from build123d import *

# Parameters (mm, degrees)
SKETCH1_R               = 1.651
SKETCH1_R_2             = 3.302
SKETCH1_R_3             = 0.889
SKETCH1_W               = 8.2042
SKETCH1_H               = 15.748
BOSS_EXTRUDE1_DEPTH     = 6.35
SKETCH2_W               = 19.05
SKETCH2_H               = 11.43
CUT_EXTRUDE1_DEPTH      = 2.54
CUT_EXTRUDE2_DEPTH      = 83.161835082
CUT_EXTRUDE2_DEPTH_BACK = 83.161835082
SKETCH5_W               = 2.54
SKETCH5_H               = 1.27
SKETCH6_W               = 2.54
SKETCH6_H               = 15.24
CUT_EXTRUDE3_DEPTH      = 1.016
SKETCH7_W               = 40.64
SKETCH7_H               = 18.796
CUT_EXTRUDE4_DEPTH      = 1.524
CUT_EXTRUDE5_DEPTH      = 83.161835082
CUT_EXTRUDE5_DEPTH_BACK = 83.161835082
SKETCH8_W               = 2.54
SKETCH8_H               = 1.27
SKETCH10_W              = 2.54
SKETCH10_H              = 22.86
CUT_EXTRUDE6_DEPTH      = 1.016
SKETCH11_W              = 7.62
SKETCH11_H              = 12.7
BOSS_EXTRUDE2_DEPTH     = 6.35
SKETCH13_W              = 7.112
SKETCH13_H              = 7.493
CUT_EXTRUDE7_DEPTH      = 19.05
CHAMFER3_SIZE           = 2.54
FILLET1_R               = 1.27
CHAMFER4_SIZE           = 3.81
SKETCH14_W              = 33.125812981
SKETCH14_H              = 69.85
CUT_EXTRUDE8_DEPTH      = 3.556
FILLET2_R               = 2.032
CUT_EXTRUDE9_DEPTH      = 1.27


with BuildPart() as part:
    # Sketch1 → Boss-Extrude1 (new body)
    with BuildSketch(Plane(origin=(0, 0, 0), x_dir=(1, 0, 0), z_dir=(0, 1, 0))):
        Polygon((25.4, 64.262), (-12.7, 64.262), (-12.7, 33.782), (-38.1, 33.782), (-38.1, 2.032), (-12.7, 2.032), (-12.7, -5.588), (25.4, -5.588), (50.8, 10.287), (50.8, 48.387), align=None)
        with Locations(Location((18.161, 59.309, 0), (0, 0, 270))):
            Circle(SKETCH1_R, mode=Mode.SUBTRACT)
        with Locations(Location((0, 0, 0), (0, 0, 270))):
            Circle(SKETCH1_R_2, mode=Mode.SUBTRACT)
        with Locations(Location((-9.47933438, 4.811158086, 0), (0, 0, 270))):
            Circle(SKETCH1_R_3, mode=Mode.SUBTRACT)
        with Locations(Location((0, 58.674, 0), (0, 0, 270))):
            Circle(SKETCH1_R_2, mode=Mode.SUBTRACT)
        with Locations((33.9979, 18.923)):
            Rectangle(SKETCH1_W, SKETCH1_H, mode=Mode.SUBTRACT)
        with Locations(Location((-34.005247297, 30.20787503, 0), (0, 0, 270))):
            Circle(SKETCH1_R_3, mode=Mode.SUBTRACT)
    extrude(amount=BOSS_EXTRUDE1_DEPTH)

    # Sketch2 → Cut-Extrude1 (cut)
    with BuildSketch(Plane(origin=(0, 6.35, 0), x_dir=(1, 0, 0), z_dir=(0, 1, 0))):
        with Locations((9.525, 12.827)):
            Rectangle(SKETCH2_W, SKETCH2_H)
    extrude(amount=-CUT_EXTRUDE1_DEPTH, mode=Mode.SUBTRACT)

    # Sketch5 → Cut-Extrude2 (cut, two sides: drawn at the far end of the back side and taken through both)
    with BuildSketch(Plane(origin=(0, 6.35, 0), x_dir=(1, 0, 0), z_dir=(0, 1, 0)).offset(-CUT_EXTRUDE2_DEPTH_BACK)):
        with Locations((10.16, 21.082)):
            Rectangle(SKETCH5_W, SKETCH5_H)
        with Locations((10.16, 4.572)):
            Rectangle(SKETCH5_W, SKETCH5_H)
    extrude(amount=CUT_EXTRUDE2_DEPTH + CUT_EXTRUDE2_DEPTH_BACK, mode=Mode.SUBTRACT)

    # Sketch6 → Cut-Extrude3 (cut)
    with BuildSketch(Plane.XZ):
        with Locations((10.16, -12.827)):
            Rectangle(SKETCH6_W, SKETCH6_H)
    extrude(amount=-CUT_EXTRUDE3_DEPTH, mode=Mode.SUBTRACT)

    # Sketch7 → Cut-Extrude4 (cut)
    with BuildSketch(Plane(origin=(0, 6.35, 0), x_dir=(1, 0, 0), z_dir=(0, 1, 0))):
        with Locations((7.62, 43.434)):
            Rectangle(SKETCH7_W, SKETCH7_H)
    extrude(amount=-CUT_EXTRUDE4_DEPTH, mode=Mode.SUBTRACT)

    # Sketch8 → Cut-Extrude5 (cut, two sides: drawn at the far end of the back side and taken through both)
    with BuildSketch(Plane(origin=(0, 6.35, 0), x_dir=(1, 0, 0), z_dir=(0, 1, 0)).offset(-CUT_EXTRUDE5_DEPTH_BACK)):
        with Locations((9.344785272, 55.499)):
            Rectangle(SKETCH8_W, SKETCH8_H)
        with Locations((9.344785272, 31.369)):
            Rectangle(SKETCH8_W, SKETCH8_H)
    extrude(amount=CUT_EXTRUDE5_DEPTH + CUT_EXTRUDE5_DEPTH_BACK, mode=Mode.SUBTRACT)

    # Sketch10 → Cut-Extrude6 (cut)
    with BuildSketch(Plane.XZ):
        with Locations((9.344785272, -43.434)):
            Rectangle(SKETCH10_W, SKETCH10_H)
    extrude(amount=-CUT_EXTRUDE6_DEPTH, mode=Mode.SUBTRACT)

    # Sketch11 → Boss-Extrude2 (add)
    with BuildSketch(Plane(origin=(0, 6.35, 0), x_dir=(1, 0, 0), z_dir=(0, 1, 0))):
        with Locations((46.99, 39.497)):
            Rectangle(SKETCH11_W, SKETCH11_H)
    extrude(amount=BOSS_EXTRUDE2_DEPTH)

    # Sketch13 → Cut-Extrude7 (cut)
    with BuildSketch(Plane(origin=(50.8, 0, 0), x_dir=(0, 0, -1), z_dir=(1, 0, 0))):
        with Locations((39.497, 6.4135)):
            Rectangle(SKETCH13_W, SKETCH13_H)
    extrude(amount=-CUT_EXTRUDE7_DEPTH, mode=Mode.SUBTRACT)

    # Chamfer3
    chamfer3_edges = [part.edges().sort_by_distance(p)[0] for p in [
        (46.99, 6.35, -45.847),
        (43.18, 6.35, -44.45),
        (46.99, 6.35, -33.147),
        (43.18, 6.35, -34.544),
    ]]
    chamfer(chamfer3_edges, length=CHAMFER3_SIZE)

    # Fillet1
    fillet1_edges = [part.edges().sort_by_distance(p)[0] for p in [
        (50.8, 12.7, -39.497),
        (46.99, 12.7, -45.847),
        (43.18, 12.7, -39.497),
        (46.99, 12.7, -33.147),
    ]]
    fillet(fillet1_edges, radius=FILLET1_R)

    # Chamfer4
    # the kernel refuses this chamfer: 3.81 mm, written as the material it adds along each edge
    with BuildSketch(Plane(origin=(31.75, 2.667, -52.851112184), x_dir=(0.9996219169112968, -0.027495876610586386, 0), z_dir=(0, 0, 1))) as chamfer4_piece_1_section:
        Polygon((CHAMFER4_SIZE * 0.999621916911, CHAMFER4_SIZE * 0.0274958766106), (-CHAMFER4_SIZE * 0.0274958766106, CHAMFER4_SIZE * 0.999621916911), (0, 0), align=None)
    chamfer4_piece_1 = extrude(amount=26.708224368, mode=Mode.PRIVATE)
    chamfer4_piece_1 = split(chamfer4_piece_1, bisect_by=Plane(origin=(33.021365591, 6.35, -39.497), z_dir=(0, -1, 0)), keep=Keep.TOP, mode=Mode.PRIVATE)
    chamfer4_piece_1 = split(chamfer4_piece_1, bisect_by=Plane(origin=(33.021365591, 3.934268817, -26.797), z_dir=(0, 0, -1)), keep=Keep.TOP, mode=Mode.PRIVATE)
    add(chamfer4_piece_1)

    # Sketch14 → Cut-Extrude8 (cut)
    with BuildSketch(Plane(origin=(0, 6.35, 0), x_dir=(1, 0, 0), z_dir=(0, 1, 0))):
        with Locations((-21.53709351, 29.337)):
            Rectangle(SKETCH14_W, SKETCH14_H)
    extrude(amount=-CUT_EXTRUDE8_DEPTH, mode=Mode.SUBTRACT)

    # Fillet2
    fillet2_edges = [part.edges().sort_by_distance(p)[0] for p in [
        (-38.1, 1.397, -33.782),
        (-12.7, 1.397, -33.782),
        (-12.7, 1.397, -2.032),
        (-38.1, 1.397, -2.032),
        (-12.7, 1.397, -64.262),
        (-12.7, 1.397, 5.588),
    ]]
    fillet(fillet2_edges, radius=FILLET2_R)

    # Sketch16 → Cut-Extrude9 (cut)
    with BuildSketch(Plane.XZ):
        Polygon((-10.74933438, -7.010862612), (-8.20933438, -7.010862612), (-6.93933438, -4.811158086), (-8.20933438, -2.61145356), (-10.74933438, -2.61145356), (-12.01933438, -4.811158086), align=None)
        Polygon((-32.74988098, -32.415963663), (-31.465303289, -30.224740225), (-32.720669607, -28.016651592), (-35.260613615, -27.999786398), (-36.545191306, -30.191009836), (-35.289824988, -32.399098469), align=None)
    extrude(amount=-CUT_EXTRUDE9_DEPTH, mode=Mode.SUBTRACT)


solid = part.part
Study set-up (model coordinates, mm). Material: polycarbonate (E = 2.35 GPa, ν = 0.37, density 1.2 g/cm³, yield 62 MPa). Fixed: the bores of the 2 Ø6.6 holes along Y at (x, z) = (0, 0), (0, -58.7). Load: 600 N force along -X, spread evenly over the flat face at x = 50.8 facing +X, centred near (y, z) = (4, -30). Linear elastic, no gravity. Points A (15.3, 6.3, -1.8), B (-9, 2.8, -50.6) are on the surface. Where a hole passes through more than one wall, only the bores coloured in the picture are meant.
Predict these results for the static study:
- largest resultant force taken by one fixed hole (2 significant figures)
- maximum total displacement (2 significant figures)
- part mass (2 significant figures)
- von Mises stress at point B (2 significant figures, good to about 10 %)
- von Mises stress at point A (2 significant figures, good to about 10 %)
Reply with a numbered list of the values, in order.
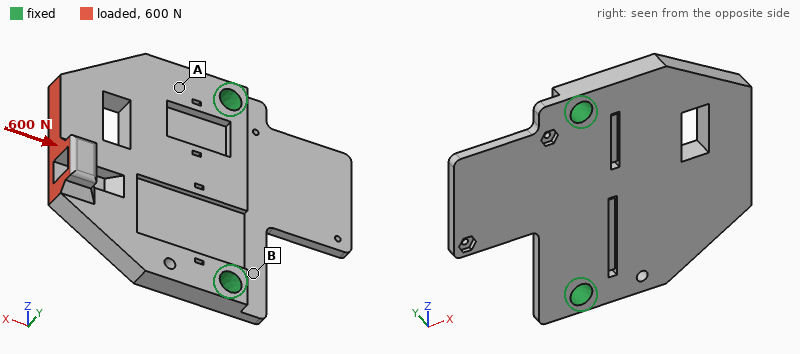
1. 320 N
2. 0.48 mm
3. 28 g
4. 1.6 MPa
5. 4.8 MPa
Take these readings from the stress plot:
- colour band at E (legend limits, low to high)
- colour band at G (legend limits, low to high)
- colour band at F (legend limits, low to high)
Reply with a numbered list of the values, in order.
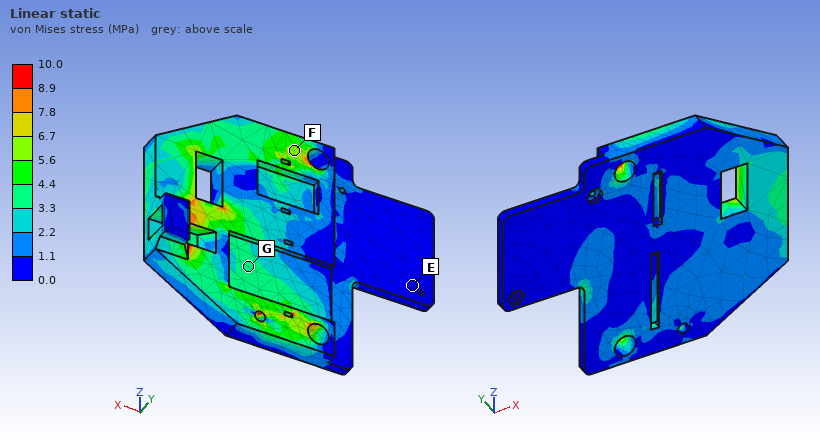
1. 0.0 to 1.1 MPa
2. 3.3 to 4.4 MPa
3. 5.6 to 6.7 MPa
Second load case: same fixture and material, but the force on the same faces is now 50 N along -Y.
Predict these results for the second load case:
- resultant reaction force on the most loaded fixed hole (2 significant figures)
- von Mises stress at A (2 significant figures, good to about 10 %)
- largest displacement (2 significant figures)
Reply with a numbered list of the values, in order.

1. 26 N
2. 6.9 MPa
3. 1.2 mm
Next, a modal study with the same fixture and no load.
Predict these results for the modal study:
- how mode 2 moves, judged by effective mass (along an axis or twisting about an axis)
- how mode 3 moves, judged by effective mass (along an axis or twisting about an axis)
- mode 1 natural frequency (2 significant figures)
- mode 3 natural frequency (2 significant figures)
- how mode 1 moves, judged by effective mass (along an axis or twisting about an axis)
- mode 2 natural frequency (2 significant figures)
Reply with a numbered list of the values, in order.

1. along Y
2. twisting about X
3. 470 Hz
4. 1300 Hz
5. along Y
6. 570 Hz
